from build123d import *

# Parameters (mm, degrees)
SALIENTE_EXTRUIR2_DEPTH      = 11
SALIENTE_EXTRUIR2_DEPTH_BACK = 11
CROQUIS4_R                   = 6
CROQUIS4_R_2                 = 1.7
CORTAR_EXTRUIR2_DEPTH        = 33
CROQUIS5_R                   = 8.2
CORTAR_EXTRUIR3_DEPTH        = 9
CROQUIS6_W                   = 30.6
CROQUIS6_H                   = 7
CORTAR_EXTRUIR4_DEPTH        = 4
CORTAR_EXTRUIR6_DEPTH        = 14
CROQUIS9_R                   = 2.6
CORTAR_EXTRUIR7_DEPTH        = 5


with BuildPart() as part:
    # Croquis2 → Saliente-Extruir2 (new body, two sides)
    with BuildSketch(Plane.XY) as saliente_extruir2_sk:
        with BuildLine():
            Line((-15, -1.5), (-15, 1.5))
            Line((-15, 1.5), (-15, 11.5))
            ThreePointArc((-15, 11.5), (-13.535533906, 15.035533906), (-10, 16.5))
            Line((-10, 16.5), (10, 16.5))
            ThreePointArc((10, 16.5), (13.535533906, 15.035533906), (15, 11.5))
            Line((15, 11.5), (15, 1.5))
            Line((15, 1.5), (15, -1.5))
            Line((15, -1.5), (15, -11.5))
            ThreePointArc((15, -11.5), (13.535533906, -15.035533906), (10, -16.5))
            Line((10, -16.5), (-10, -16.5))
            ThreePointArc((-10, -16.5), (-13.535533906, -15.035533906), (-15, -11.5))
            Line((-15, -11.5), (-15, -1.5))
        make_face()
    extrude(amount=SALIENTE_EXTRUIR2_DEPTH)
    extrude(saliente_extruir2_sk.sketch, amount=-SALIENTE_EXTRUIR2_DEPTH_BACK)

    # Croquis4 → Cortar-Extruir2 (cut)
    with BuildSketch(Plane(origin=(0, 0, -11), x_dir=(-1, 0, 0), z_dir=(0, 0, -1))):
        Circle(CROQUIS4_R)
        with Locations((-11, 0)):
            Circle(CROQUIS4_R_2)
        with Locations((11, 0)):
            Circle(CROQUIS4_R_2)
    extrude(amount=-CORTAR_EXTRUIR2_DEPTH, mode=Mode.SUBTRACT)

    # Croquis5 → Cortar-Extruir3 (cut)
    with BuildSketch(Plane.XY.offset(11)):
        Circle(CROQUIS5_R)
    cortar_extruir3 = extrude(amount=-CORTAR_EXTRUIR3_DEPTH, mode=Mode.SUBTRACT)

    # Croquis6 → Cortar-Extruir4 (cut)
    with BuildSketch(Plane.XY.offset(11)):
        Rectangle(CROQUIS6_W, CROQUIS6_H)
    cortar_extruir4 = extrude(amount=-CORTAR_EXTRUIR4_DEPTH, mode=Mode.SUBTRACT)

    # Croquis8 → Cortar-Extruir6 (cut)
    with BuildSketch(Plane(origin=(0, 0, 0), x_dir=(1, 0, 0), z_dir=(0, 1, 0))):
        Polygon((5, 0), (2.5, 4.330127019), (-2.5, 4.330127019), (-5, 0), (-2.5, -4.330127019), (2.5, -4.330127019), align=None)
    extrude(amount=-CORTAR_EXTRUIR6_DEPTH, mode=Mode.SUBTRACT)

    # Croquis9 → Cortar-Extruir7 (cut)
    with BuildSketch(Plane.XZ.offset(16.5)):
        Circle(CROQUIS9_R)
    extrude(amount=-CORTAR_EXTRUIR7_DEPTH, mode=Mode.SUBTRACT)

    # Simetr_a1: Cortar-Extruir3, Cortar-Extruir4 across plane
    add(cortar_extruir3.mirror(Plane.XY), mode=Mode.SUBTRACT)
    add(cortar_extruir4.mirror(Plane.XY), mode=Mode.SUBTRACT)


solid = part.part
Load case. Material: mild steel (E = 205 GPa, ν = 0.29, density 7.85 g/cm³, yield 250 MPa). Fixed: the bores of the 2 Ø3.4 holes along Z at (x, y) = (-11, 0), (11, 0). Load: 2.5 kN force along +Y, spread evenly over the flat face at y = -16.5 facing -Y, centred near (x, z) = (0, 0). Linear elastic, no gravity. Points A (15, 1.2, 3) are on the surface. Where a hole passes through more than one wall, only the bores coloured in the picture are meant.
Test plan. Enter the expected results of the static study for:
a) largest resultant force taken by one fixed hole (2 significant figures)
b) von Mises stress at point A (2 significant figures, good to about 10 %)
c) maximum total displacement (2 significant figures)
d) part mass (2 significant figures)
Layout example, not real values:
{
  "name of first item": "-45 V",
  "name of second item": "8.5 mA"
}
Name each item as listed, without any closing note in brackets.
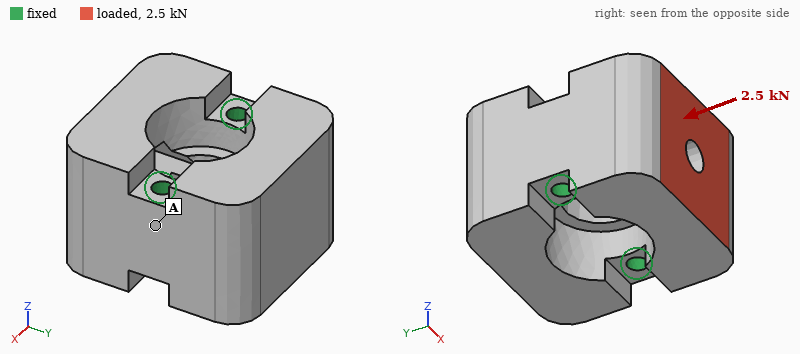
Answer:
{
  "largest resultant force taken by one fixed hole": "1.3 kN",
  "von Mises stress at point A": "4.1 MPa",
  "maximum total displacement": "1.4 µm",
  "part mass": "120 g"
}
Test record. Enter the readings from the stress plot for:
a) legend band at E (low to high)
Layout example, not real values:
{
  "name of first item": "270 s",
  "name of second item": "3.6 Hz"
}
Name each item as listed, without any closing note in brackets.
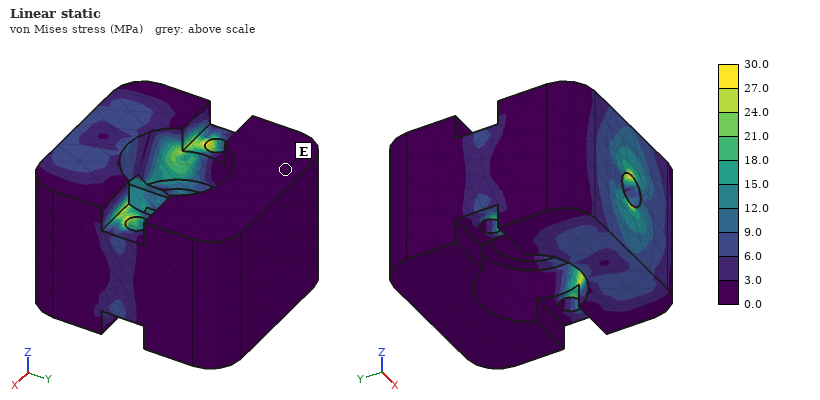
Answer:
{
  "legend band at E": "0.0 to 3.0 MPa"
}
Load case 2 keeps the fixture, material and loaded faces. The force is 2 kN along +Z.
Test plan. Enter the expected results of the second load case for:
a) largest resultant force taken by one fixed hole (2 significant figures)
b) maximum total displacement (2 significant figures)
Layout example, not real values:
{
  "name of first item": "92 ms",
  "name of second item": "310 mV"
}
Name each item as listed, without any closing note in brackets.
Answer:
{
  "largest resultant force taken by one fixed hole": "1.0 kN",
  "maximum total displacement": "6.6 µm"
}
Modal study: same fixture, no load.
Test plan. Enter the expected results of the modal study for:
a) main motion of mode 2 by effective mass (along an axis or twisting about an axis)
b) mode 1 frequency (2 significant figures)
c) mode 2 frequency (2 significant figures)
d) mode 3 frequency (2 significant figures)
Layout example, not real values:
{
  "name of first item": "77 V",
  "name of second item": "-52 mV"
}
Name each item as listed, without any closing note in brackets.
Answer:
{
  "main motion of mode 2 by effective mass": "along Z",
  "mode 1 frequency": "18 kHz",
  "mode 2 frequency": "19 kHz",
  "mode 3 frequency": "24 kHz"
}
